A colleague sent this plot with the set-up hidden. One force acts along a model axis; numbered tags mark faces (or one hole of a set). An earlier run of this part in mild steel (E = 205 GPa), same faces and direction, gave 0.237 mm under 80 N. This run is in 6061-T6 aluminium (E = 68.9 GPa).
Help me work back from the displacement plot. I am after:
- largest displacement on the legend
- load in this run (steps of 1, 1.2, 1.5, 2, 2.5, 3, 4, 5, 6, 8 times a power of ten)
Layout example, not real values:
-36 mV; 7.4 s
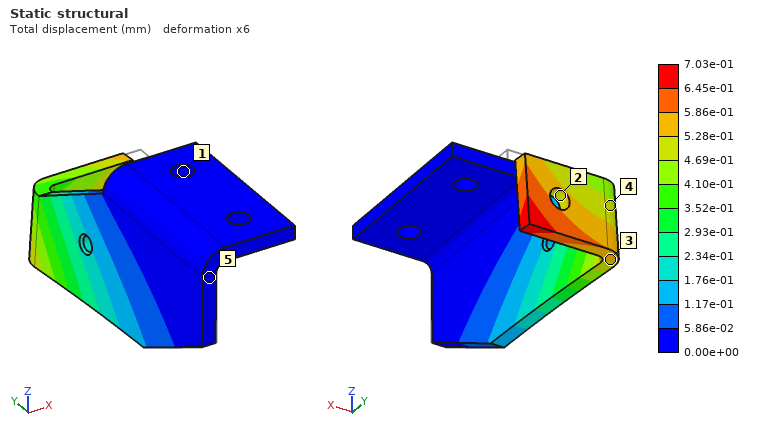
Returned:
7.03e-01 mm; 80 N
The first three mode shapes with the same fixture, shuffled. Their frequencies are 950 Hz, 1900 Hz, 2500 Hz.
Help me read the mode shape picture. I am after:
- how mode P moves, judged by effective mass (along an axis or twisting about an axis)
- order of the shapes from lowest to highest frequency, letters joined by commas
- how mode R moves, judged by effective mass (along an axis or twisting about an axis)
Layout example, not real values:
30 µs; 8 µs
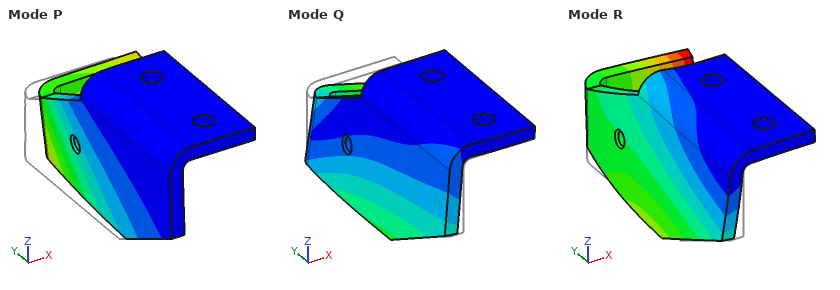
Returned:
along X; P, Q, R; along Z
